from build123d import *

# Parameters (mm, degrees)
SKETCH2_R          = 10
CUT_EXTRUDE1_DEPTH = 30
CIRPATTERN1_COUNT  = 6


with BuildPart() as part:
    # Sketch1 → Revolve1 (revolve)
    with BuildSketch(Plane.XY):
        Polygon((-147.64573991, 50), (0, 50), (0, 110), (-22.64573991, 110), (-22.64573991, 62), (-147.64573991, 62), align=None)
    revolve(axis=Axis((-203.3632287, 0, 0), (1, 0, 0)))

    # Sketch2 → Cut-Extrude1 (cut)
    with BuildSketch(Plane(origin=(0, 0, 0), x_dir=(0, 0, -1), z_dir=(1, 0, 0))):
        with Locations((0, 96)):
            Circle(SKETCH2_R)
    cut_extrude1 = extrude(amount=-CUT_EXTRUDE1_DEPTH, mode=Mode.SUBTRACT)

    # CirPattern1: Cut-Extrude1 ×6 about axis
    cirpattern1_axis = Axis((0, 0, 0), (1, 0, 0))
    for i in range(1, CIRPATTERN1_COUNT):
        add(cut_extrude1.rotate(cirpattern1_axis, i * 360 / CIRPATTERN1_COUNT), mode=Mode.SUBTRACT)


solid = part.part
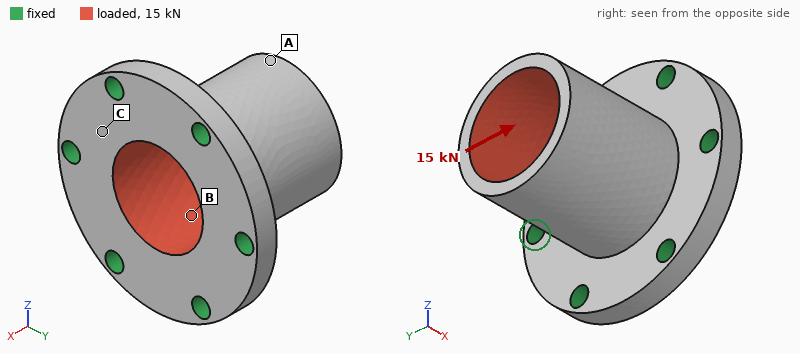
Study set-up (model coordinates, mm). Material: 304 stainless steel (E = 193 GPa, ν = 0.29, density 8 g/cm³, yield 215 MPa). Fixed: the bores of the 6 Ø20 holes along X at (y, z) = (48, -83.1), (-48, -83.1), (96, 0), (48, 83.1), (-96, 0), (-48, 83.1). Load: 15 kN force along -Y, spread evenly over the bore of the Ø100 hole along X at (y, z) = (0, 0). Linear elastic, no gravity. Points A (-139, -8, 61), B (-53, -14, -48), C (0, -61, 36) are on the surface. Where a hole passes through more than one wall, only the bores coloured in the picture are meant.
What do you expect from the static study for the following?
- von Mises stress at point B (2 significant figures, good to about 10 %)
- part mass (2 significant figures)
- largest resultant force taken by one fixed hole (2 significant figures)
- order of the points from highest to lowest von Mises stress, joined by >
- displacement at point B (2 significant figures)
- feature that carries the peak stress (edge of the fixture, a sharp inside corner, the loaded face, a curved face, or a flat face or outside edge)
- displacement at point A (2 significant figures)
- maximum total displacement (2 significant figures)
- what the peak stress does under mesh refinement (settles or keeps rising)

9.2 MPa
9.3 kg
5.3 kN
B > C > A
4.8 µm
edge of the fixture
14 µm
17 µm
keeps rising
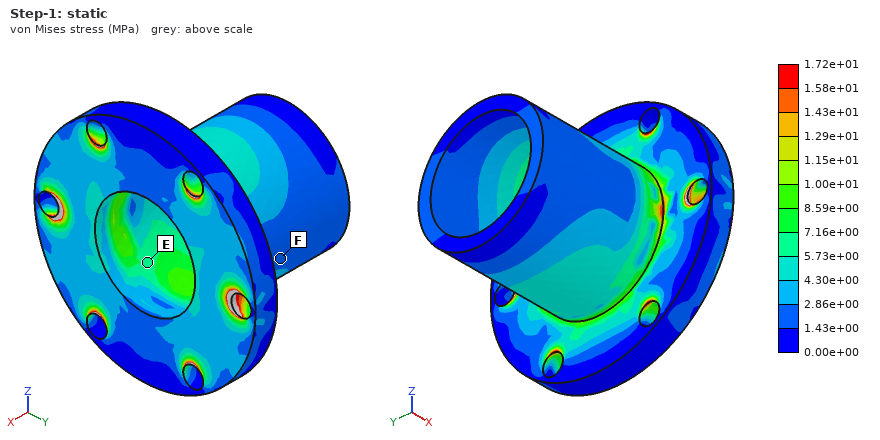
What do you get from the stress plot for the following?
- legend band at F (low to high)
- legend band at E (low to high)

1.43e+00 to 2.86e+00 MPa
5.73e+00 to 7.16e+00 MPa
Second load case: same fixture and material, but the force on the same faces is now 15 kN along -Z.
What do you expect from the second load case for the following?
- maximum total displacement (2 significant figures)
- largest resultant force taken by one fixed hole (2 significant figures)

17 µm
4.7 kN
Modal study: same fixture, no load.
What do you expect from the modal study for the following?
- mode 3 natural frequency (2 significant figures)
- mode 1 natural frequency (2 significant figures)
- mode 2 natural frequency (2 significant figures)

2900 Hz
2500 Hz
2500 Hz
